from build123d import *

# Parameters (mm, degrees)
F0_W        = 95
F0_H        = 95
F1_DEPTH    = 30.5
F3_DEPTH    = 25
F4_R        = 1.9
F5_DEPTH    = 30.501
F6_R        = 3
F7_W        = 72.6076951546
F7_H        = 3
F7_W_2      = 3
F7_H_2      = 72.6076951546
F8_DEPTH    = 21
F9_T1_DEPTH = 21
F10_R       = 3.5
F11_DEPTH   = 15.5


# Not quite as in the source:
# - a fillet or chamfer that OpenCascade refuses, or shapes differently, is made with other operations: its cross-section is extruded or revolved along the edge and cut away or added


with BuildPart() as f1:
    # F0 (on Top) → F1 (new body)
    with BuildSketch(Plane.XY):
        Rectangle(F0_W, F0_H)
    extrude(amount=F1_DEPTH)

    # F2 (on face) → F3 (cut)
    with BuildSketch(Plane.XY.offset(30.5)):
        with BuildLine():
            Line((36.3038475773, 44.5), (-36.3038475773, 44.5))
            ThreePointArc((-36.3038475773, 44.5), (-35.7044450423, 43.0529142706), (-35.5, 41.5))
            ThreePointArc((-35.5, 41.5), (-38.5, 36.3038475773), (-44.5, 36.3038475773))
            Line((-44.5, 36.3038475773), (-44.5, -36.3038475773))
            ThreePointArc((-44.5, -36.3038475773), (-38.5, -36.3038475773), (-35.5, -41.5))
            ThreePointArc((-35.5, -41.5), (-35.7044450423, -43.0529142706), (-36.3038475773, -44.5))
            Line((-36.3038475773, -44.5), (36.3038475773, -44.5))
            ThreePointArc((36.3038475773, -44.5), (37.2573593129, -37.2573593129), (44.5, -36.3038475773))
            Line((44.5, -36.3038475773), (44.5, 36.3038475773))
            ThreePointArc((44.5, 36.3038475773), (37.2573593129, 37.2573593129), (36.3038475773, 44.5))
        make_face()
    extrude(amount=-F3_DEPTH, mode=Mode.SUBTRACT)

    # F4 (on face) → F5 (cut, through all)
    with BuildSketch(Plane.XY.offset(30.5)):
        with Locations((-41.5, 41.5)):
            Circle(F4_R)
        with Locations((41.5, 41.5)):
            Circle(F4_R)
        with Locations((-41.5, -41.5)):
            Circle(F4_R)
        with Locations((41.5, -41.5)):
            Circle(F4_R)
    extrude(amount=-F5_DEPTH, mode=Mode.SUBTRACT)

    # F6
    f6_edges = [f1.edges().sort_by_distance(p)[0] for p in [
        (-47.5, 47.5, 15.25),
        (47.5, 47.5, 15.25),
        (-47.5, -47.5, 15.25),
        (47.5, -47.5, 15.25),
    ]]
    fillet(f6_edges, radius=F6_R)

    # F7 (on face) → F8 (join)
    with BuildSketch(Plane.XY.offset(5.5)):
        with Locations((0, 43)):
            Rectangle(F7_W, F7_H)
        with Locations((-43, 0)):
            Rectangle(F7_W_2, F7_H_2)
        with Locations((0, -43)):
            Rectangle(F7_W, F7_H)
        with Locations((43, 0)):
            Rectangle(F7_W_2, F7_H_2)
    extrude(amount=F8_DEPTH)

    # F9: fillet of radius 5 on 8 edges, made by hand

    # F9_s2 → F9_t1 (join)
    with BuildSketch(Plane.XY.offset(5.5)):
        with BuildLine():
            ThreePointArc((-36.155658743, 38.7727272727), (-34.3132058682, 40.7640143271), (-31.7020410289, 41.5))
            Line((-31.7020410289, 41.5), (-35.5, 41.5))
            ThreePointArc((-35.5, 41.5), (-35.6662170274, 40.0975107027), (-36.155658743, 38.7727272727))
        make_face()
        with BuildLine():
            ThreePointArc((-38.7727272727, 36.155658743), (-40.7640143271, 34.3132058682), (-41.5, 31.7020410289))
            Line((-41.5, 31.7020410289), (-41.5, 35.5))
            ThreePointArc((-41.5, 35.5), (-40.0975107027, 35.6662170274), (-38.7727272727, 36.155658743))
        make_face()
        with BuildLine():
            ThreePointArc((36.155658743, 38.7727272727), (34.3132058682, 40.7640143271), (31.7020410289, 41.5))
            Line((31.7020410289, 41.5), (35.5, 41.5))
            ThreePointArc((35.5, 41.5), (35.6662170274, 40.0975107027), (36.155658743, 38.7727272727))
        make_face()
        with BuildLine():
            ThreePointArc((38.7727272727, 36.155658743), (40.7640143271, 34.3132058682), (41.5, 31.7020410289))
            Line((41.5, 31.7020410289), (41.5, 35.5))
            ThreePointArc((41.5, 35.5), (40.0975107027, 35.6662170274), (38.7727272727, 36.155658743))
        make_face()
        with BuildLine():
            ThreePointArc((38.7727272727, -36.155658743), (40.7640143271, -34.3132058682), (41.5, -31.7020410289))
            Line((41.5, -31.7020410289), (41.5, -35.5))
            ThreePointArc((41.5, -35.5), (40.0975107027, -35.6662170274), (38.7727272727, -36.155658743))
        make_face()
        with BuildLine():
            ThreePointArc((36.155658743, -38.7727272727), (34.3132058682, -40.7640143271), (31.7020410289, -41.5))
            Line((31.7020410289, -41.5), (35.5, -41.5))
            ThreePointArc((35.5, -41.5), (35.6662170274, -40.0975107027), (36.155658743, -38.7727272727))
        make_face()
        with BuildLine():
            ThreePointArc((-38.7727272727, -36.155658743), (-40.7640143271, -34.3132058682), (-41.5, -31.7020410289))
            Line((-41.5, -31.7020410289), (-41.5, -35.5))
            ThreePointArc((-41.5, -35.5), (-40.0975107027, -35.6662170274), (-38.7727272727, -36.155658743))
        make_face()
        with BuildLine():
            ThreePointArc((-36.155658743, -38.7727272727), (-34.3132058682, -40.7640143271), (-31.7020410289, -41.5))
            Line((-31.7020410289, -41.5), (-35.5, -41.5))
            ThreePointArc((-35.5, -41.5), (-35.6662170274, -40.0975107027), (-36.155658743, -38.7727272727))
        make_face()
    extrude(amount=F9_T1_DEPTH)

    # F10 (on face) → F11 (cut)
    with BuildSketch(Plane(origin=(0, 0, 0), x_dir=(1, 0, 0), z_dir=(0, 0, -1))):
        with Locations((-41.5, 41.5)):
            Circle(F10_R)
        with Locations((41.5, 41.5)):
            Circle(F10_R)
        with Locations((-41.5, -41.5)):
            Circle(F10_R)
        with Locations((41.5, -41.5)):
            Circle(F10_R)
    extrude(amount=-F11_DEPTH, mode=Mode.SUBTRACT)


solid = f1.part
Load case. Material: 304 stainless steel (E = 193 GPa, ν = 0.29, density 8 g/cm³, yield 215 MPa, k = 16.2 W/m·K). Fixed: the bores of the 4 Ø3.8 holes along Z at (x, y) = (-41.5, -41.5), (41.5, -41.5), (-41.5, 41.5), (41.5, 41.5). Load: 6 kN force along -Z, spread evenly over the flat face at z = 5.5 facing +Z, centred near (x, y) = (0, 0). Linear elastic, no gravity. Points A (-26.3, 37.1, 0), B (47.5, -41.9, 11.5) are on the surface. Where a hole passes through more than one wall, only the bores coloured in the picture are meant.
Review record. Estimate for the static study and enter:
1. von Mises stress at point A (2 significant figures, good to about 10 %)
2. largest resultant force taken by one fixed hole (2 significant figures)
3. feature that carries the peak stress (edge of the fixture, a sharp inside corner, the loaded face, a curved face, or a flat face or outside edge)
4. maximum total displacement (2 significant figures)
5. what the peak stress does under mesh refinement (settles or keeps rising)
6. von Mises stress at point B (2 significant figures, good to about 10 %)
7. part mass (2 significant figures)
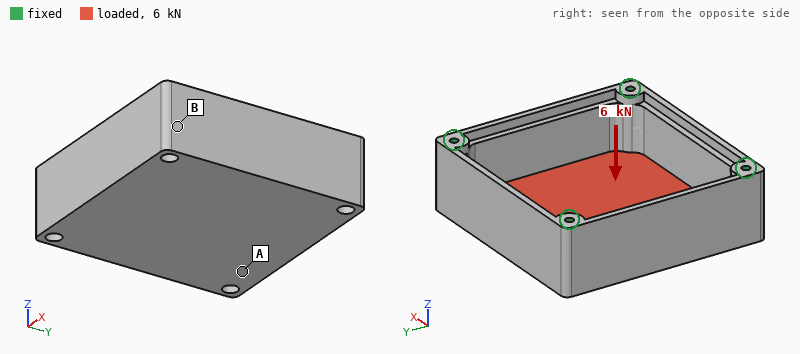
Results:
22 MPa
1.9 kN
edge of the fixture
40 µm
keeps rising
5.1 MPa
800 g
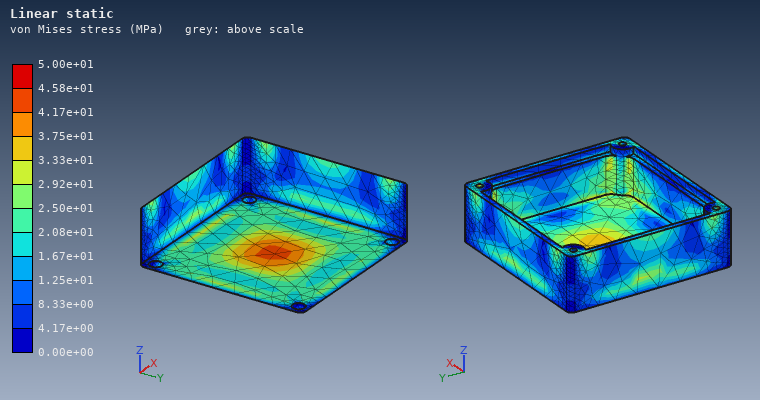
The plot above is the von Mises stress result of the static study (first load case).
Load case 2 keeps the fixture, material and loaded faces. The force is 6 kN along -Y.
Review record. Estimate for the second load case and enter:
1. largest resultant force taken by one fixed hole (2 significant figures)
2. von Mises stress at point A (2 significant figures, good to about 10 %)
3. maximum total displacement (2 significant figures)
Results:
1.6 kN
7.6 MPa
4.8 µm
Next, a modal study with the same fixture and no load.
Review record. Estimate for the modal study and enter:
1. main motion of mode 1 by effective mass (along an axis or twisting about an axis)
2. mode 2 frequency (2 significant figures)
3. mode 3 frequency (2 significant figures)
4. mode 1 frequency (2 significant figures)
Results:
along Z
7200 Hz
7200 Hz
4300 Hz
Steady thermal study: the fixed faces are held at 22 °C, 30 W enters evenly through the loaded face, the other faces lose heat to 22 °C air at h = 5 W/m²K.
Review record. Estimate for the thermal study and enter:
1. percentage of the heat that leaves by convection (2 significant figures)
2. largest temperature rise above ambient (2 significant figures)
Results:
14 %
60 K
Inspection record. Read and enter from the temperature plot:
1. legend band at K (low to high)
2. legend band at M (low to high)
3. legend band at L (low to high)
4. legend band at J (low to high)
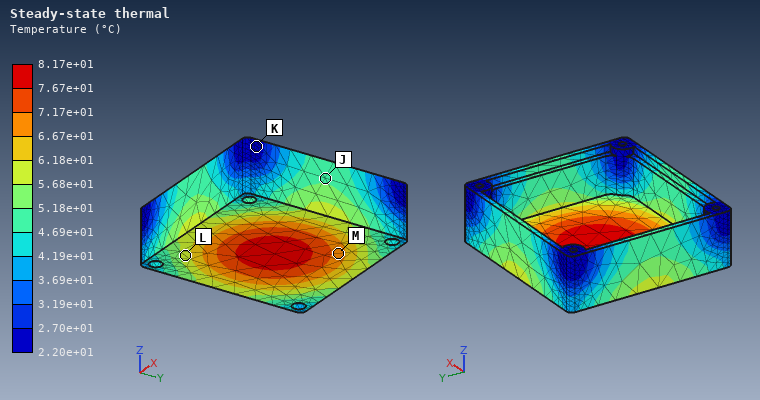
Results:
2.20e+01 to 2.70e+01 °C
6.67e+01 to 7.17e+01 °C
5.68e+01 to 6.18e+01 °C
4.69e+01 to 5.18e+01 °C
